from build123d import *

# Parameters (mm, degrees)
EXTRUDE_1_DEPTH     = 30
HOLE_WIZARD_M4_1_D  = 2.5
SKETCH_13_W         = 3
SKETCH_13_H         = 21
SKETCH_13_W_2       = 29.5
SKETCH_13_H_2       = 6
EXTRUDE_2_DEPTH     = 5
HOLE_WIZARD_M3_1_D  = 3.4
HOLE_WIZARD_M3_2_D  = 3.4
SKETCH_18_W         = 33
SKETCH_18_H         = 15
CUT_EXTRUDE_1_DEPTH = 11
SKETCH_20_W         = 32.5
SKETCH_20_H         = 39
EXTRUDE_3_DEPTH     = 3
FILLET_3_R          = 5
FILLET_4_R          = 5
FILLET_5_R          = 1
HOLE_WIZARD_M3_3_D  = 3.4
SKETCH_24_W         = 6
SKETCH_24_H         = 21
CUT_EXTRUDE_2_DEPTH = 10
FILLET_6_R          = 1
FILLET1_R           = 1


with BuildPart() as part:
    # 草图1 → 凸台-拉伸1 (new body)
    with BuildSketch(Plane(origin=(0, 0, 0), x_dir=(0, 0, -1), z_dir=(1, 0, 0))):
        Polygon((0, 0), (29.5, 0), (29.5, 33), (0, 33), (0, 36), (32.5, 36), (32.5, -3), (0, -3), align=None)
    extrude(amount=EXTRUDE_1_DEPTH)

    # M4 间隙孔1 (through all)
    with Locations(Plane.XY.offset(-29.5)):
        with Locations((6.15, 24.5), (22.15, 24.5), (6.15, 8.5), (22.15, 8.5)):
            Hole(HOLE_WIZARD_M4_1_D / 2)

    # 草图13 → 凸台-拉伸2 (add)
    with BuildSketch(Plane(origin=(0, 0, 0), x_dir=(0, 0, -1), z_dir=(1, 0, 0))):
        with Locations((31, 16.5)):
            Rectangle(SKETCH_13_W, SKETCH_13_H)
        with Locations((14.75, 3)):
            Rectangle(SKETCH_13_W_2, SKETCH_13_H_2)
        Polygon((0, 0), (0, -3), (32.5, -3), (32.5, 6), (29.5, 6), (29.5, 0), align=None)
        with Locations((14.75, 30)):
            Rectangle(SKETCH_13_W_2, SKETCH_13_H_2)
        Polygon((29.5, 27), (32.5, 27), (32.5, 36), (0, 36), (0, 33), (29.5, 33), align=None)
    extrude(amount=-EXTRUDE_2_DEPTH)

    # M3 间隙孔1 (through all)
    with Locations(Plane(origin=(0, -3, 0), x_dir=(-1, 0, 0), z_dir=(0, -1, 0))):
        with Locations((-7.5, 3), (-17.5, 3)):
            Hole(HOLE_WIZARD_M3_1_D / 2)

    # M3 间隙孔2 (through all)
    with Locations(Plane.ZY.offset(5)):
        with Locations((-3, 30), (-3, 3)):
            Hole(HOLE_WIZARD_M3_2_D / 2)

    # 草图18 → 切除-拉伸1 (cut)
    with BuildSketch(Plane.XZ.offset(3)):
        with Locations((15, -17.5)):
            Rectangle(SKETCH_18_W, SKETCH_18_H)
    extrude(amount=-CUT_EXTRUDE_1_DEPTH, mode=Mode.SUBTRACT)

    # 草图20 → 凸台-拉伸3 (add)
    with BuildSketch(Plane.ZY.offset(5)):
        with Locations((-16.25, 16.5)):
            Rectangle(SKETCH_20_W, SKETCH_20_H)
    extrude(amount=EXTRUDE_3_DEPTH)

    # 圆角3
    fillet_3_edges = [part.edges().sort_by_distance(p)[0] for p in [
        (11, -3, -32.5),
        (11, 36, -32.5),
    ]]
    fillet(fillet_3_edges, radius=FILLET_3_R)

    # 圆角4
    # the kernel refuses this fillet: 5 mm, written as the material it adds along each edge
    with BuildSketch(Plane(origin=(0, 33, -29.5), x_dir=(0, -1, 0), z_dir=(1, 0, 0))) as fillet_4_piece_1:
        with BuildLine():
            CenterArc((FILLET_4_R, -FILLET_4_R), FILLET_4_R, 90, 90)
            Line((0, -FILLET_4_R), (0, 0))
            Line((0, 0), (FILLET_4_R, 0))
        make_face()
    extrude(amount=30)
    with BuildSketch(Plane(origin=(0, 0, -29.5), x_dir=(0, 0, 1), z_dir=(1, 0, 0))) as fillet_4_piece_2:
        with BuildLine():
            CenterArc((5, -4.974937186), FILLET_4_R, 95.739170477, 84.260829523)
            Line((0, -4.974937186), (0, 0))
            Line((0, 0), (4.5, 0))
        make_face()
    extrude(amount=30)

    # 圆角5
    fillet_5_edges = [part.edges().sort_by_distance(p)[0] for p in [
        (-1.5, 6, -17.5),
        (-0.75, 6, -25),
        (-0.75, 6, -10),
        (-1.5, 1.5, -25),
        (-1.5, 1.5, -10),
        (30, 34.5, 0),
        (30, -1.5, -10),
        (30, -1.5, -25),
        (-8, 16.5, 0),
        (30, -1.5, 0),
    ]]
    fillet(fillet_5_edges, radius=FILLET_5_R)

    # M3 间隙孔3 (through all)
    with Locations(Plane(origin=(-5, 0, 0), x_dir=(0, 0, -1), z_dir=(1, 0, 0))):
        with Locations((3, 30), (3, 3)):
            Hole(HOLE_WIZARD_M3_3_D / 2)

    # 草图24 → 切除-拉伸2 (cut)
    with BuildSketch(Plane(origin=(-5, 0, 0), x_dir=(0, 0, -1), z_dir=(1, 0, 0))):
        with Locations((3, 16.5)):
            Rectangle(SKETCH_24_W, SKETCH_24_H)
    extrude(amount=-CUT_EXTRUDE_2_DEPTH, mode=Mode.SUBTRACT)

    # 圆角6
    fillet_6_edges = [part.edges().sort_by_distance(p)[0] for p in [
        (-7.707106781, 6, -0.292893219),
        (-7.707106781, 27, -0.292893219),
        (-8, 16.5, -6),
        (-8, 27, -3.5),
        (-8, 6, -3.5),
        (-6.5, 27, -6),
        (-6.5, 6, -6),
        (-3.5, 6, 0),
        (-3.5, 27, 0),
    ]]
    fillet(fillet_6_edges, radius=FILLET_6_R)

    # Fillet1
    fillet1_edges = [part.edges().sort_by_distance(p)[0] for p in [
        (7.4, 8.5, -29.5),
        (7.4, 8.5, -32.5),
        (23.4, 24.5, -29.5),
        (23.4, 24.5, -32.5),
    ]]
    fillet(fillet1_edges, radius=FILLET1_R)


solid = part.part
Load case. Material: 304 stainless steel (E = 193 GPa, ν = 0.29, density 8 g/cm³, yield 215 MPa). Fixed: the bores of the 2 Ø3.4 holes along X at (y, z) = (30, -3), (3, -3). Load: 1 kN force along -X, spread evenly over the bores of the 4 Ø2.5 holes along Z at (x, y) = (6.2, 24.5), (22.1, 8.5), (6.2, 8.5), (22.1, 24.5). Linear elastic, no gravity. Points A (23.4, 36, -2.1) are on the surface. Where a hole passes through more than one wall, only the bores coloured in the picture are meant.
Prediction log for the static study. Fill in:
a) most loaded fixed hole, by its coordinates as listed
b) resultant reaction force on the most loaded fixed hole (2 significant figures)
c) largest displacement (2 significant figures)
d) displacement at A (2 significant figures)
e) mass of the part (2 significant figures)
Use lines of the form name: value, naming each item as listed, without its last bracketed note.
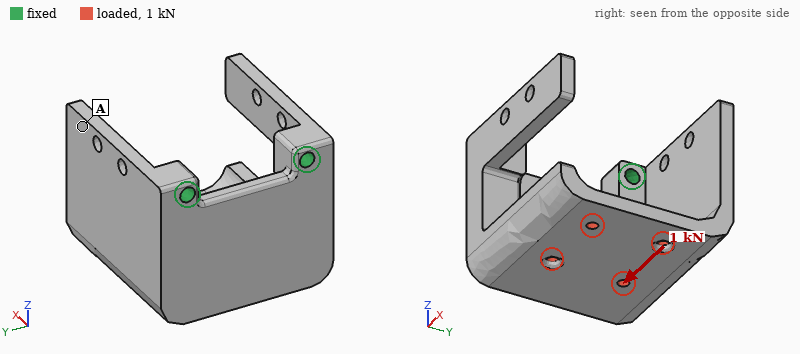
most loaded fixed hole, by its coordinates as listed: (30, -3)
resultant reaction force on the most loaded fixed hole: 580 N
largest displacement: 88 µm
displacement at A: 37 µm
mass of the part: 110 g
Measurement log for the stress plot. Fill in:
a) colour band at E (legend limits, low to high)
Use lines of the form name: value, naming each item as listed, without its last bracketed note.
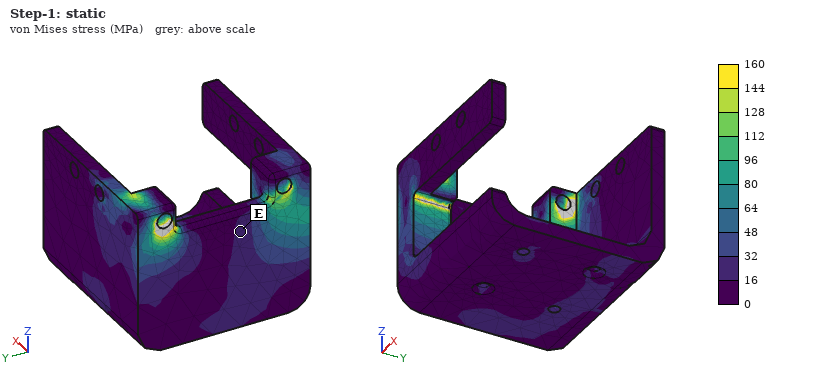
colour band at E: 16 to 32 MPa
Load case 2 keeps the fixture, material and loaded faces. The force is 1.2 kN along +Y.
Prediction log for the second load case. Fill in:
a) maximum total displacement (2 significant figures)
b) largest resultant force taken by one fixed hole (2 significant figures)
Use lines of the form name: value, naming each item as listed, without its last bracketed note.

maximum total displacement: 98 µm
largest resultant force taken by one fixed hole: 1.2 kN
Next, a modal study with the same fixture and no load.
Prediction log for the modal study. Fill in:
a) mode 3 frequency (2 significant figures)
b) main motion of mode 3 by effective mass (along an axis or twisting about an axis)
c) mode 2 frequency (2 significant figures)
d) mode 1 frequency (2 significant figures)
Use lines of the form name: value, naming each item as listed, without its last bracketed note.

mode 3 frequency: 2800 Hz
main motion of mode 3 by effective mass: along Y
mode 2 frequency: 2500 Hz
mode 1 frequency: 2300 Hz
